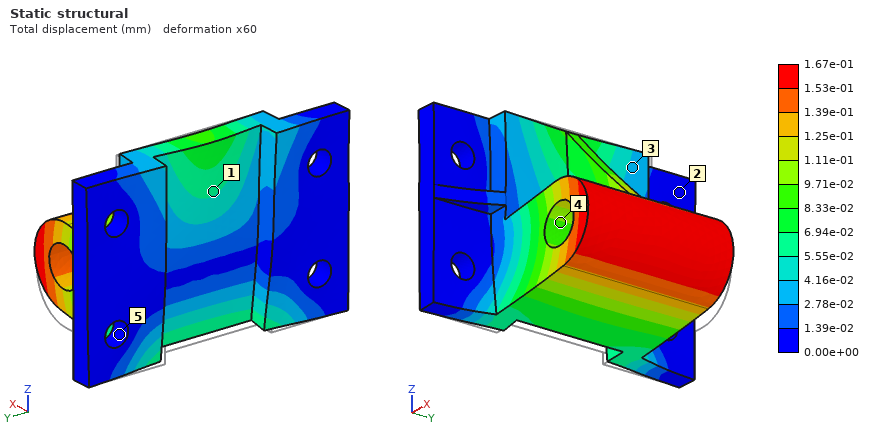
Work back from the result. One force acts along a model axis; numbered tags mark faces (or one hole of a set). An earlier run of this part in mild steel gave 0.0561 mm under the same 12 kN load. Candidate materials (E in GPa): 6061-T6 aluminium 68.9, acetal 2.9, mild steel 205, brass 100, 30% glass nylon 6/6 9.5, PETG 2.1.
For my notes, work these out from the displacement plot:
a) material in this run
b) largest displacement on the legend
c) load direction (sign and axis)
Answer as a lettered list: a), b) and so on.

a) 6061-T6 aluminium
b) 1.67e-01 mm
c) +Z
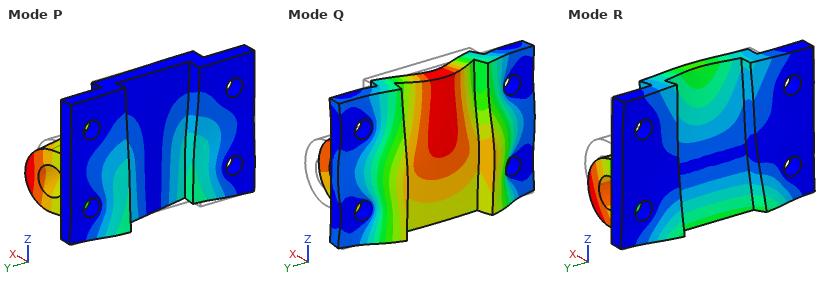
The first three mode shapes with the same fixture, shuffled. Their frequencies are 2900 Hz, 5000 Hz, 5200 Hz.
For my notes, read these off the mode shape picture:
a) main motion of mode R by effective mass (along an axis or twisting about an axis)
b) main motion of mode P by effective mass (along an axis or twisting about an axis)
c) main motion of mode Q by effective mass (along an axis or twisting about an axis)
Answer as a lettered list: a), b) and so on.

a) along Z
b) along Y
c) along X
